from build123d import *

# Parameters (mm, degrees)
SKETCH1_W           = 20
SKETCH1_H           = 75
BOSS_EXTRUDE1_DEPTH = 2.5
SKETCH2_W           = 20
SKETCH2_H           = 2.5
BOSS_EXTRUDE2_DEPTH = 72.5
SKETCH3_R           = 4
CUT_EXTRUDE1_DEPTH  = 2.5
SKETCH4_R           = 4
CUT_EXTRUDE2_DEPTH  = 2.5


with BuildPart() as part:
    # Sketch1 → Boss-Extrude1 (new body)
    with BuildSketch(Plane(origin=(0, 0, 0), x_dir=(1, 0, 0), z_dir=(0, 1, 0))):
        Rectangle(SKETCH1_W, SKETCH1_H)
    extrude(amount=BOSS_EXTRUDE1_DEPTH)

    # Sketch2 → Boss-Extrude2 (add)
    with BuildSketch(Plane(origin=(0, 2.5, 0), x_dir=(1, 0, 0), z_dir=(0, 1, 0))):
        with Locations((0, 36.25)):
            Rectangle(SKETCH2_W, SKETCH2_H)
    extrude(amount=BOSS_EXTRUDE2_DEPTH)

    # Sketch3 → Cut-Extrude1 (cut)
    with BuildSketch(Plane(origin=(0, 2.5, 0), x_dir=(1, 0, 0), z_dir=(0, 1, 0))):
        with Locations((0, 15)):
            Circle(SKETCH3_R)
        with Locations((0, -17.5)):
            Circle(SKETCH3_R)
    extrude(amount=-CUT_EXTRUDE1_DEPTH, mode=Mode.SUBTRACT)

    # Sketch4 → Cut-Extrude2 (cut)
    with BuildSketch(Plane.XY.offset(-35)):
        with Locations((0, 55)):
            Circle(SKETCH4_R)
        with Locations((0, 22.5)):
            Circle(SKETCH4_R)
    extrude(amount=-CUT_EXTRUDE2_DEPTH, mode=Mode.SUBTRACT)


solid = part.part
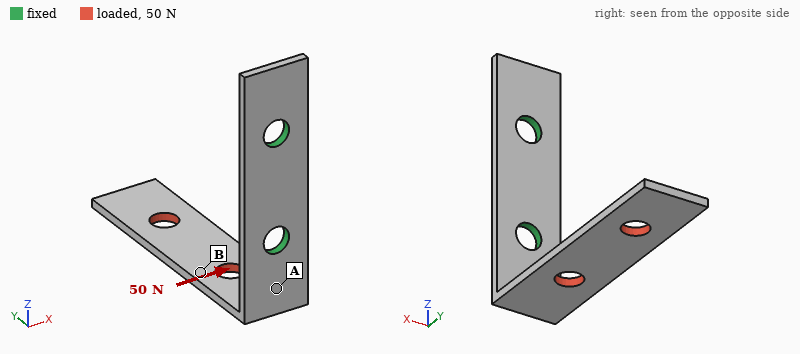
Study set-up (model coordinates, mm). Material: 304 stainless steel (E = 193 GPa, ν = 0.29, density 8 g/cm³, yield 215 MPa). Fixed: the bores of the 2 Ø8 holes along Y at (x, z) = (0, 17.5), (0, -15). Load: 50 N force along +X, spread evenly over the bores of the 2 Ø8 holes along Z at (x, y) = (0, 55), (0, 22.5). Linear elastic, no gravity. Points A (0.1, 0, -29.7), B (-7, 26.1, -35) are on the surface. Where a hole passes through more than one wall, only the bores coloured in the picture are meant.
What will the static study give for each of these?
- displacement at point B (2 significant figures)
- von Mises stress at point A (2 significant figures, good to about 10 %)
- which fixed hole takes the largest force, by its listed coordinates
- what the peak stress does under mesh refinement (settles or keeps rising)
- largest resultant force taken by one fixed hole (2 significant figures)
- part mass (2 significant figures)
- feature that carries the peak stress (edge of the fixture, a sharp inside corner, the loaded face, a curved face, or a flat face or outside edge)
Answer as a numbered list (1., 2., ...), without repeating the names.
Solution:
1. 0.097 mm
2. 67 MPa
3. (0, -15)
4. keeps rising
5. 60 N
6. 55 g
7. edge of the fixture
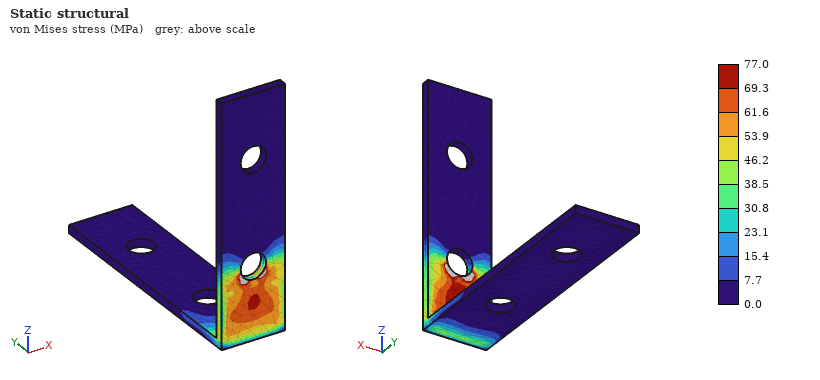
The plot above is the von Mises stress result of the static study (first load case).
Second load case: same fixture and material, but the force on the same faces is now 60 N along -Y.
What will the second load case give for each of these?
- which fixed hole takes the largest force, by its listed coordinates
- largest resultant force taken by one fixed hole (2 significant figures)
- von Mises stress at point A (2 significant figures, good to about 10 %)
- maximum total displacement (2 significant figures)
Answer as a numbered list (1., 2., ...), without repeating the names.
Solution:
1. (0, -15)
2. 60 N
3. 16 MPa
4. 0.15 mm
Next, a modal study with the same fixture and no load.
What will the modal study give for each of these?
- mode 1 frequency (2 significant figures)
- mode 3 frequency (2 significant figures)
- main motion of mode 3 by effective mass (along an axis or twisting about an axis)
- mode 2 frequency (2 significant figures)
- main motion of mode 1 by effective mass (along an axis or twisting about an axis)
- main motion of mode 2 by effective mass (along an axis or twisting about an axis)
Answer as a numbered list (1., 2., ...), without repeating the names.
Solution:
1. 260 Hz
2. 1500 Hz
3. along Y
4. 500 Hz
5. along Z
6. along X
